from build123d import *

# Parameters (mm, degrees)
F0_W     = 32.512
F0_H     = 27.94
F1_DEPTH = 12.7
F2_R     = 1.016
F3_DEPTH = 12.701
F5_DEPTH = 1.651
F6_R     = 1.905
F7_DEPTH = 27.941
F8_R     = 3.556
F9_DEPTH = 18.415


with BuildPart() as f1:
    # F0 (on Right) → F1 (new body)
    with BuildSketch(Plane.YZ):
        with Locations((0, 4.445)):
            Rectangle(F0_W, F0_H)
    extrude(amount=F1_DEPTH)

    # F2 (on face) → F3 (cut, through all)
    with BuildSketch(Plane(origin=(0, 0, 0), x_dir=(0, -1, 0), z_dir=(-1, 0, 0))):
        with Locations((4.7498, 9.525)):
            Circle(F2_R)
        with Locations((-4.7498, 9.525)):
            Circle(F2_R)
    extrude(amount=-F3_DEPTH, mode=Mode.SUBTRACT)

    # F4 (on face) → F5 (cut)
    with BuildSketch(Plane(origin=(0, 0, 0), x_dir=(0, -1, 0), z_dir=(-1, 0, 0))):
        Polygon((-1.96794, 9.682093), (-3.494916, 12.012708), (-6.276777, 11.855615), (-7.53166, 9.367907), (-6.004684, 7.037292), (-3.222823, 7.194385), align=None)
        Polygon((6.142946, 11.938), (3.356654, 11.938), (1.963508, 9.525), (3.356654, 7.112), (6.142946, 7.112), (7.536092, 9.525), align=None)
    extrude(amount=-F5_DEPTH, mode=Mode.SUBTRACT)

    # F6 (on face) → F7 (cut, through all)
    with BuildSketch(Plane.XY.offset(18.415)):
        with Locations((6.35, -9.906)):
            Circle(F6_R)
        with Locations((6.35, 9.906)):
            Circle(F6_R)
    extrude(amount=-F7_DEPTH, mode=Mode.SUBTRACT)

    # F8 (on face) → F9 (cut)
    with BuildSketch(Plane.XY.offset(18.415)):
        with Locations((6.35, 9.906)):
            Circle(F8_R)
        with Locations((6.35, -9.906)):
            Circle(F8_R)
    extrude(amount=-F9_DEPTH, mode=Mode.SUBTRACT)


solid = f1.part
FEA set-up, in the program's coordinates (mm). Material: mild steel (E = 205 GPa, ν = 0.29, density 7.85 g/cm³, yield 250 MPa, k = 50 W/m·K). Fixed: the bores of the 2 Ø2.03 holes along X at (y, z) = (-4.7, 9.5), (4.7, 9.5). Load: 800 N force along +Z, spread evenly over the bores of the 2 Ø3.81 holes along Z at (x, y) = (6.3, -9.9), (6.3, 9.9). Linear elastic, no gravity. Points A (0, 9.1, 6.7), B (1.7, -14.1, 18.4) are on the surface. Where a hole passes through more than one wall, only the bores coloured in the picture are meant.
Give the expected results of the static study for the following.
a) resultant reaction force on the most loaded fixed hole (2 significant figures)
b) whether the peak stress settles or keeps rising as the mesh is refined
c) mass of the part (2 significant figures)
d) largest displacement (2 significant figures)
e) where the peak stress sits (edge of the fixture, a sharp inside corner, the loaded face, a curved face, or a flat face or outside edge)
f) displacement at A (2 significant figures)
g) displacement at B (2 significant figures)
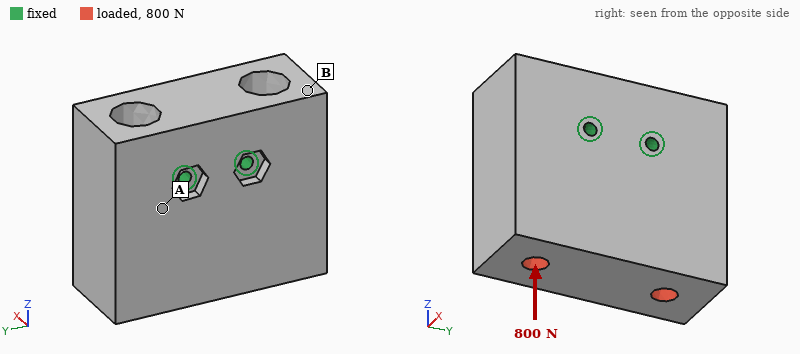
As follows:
400 N
keeps rising
76 g
0.50 µm
edge of the fixture
0.22 µm
0.28 µm
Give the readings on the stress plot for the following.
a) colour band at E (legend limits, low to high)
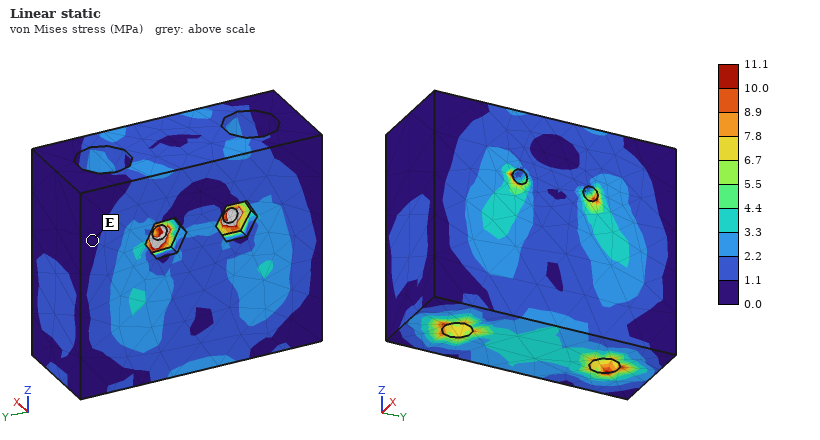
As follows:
0.0 to 1.1 MPa
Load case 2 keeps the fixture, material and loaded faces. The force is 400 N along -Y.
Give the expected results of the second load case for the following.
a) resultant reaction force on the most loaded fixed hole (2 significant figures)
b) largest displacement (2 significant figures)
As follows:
570 N
1.2 µm
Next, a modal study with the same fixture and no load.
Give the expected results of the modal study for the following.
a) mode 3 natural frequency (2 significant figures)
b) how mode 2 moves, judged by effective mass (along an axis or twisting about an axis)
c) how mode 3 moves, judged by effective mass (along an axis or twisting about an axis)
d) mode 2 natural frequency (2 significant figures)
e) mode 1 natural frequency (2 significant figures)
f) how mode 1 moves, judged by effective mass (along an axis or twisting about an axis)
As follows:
18 kHz
along Y
twisting about Z
16 kHz
15 kHz
along X
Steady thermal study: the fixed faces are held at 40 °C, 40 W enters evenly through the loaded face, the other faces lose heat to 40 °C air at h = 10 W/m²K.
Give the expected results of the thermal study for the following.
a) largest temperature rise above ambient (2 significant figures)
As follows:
50 K
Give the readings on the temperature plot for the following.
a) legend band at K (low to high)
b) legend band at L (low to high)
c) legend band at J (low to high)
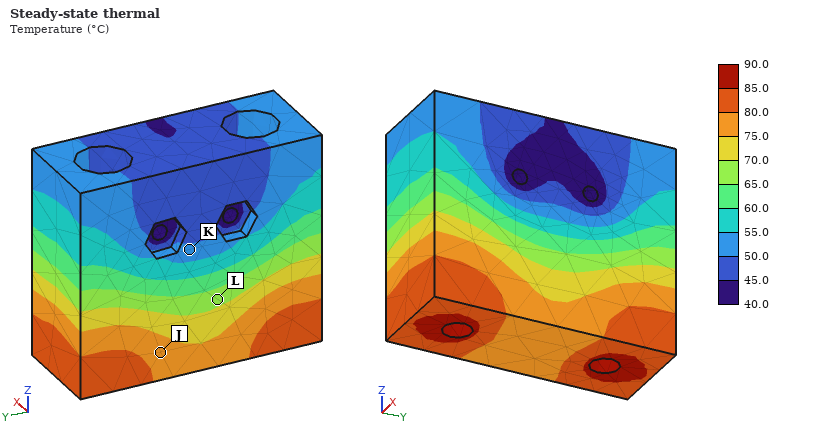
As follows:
50.0 to 55.0 °C
65.0 to 70.0 °C
75.0 to 80.0 °C
